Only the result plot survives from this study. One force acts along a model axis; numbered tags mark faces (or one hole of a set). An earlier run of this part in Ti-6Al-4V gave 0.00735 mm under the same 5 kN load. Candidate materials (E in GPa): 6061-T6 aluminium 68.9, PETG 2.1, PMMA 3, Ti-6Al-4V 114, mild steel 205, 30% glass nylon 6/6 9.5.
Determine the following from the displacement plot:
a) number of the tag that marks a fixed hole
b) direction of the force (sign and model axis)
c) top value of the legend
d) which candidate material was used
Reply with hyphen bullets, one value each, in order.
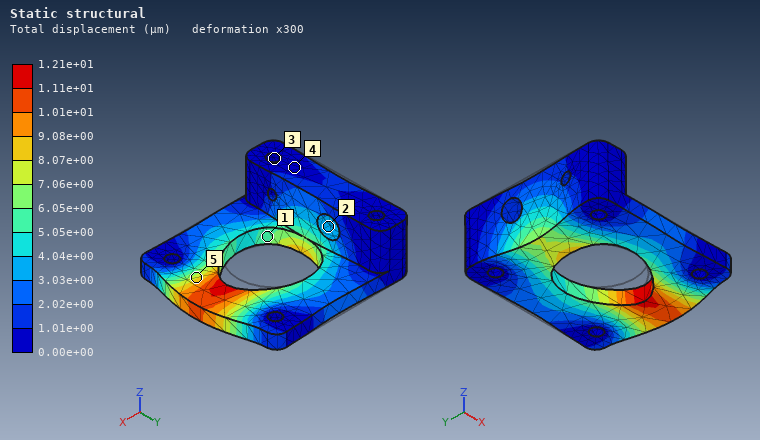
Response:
- 3
- +X
- 1.21e+01 µm
- 6061-T6 aluminium
